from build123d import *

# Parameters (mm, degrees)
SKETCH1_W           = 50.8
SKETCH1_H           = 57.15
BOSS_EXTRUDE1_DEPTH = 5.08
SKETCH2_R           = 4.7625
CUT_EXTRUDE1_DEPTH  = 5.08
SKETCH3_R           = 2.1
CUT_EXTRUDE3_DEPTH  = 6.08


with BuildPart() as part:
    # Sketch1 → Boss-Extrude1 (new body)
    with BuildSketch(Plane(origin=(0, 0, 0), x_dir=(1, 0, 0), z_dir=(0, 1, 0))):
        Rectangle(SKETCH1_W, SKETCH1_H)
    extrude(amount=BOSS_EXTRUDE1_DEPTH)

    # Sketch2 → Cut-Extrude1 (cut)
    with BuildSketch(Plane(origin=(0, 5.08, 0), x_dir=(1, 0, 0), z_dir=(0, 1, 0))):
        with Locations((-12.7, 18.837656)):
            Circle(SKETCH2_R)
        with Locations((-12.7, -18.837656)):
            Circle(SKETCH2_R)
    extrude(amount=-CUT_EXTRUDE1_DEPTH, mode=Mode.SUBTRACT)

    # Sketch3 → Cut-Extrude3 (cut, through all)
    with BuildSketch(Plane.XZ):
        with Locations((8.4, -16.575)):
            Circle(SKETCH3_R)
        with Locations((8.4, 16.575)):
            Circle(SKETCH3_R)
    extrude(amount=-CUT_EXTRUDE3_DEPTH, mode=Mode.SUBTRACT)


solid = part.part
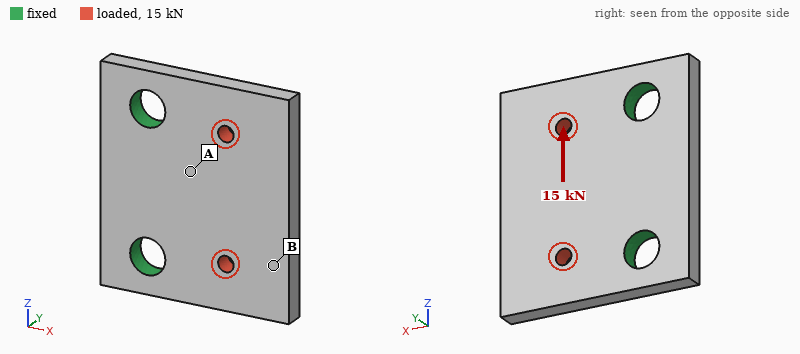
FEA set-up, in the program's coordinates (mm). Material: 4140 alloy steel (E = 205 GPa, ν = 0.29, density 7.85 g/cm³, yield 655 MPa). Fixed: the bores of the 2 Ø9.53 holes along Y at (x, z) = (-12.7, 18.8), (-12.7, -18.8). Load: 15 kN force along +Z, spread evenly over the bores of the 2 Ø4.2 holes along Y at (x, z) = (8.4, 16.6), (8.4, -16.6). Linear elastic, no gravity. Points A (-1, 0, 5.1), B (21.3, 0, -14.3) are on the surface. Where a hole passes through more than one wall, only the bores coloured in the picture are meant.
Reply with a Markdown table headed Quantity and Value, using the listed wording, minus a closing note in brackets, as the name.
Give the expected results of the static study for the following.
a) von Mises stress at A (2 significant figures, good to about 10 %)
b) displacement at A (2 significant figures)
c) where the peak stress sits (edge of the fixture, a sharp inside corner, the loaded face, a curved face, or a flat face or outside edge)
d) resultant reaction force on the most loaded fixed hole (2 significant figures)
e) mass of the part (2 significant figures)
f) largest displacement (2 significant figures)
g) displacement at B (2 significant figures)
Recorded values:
| Quantity | Value |
|---|---|
| von Mises stress at A | 100 MPa |
| displacement at A | 8.2 µm |
| where the peak stress sits | edge of the fixture |
| resultant reaction force on the most loaded fixed hole | 10.0 kN |
| mass of the part | 110 g |
| largest displacement | 22 µm |
| displacement at B | 21 µm |
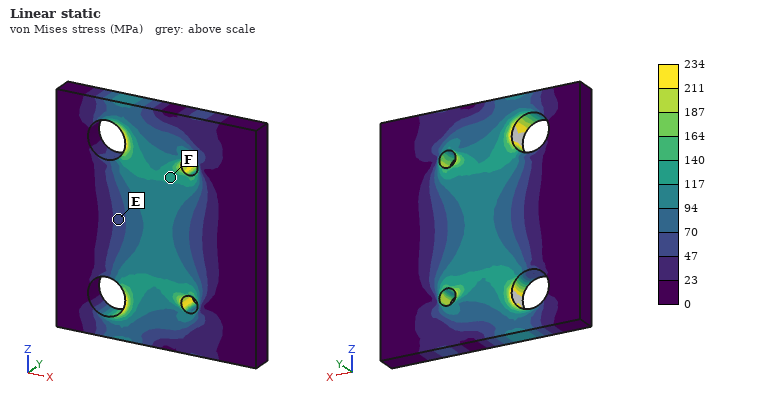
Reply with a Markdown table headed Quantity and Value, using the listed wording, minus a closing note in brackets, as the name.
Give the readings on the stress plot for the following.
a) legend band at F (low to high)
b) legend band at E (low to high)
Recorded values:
| Quantity | Value |
|---|---|
| legend band at F | 117 to 140 MPa |
| legend band at E | 47 to 70 MPa |
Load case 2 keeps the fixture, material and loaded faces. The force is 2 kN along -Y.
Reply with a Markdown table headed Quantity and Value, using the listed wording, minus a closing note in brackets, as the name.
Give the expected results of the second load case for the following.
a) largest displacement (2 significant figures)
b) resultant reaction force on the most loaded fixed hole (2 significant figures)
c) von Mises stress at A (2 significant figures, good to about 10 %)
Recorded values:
| Quantity | Value |
|---|---|
| largest displacement | 84 µm |
| resultant reaction force on the most loaded fixed hole | 1.0 kN |
| von Mises stress at A | 58 MPa |
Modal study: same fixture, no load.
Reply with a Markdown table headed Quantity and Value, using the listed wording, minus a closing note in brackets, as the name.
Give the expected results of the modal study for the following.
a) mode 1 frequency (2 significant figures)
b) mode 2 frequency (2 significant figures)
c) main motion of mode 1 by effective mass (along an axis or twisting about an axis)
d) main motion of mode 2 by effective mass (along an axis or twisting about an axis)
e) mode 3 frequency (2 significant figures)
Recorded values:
| Quantity | Value |
|---|---|
| mode 1 frequency | 3200 Hz |
| mode 2 frequency | 5800 Hz |
| main motion of mode 1 by effective mass | along Y |
| main motion of mode 2 by effective mass | twisting about X |
| mode 3 frequency | 11 kHz |
